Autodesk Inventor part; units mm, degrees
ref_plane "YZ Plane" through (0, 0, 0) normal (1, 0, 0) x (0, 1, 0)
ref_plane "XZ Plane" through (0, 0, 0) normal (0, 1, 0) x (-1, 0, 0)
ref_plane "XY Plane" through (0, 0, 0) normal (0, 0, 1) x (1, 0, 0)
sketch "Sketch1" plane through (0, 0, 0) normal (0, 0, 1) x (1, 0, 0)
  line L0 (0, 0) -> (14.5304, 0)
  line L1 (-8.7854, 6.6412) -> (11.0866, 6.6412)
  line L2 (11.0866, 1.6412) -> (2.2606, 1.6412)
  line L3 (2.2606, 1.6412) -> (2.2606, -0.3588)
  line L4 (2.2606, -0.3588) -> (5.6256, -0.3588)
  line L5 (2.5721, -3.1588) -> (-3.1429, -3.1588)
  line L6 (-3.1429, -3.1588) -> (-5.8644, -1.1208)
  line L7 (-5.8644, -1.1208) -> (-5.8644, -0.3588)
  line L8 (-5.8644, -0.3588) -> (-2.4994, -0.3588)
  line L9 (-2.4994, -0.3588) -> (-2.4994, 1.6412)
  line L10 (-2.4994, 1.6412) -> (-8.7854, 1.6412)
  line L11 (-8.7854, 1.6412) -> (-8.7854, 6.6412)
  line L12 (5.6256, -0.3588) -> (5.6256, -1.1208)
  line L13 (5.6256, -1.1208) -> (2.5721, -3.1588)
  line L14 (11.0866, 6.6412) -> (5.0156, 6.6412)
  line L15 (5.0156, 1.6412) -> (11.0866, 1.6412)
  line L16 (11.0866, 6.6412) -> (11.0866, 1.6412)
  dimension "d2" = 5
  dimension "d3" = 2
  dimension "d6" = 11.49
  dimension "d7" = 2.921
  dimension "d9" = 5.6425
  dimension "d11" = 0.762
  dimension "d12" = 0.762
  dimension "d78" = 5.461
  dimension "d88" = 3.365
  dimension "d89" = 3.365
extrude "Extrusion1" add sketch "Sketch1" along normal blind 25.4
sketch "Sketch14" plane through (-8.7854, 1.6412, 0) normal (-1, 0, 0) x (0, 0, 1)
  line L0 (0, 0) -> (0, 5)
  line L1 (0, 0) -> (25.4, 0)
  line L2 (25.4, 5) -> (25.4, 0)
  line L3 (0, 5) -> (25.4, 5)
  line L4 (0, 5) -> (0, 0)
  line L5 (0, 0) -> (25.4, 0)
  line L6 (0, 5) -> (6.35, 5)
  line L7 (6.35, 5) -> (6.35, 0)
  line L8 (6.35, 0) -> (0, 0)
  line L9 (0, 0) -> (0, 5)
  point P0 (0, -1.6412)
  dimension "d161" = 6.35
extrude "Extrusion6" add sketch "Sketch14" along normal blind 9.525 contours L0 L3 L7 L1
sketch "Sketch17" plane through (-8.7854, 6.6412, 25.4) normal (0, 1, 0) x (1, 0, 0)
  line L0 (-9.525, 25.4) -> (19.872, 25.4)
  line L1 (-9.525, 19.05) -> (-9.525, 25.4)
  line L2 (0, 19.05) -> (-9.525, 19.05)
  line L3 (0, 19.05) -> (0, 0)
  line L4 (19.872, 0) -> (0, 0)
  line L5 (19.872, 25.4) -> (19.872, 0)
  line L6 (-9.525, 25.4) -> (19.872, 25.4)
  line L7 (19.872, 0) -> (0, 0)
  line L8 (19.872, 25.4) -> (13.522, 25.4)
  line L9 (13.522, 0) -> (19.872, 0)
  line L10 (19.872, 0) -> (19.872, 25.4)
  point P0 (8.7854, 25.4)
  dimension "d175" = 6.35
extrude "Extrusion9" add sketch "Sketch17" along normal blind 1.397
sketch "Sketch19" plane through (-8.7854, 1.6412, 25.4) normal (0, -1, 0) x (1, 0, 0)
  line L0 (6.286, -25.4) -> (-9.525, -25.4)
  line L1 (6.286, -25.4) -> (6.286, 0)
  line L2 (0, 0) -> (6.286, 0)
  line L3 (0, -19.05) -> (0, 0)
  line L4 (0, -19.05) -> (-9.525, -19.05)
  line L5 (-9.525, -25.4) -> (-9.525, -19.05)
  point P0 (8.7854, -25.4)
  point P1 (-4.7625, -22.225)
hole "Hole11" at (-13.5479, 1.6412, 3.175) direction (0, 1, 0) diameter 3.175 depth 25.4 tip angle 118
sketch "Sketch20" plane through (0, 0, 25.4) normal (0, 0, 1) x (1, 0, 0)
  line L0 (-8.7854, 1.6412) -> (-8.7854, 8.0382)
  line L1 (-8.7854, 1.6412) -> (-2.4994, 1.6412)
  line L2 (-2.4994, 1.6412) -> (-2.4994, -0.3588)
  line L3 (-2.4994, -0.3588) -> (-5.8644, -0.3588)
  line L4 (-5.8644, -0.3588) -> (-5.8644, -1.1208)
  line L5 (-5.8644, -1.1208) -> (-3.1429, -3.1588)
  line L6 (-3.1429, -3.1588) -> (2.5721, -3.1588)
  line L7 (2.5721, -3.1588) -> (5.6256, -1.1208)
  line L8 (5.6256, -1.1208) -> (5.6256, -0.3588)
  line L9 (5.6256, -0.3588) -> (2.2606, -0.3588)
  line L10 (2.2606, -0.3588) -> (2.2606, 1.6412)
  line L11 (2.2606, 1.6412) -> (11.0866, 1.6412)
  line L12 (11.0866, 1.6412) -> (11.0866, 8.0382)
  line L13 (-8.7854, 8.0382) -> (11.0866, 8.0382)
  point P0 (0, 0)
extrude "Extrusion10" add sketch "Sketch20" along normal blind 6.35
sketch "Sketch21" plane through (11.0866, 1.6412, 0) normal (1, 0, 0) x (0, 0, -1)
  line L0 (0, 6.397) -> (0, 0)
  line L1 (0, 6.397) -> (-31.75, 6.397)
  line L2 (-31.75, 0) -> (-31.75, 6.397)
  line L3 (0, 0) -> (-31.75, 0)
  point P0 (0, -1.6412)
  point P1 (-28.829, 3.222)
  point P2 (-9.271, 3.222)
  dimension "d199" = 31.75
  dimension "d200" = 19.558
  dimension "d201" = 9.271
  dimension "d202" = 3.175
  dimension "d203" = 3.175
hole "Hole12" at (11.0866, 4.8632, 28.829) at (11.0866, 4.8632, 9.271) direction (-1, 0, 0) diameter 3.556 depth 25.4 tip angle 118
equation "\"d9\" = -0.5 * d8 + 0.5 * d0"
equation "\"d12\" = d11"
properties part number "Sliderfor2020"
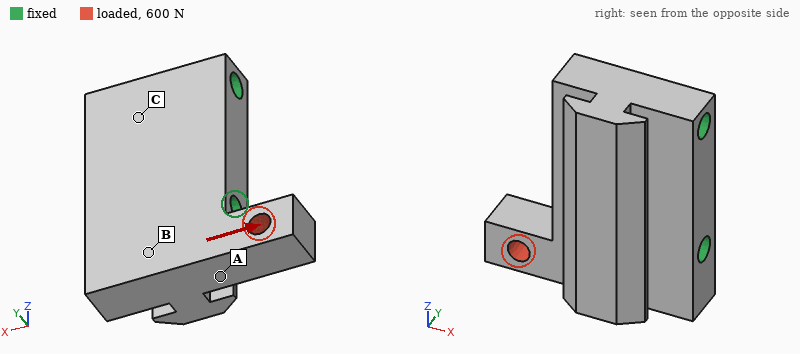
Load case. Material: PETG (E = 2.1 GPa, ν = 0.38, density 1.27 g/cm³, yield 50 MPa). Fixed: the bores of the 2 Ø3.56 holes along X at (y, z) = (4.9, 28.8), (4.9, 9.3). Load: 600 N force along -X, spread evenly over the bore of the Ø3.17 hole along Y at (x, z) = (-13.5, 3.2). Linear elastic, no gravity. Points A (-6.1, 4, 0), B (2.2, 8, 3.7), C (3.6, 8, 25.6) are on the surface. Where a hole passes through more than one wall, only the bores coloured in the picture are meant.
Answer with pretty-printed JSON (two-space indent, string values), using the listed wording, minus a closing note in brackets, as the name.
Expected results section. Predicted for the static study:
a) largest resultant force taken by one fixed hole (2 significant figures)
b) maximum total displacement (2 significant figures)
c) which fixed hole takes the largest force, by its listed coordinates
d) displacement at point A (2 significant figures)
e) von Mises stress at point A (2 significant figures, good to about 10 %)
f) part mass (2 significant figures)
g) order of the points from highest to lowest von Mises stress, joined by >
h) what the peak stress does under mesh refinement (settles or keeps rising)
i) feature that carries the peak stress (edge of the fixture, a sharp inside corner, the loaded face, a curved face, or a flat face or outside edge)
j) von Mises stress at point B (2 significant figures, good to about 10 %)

{
  "largest resultant force taken by one fixed hole": "610 N",
  "maximum total displacement": "0.19 mm",
  "which fixed hole takes the largest force, by its listed coordinates": "(4.9, 9.3)",
  "displacement at point A": "0.076 mm",
  "von Mises stress at point A": "17 MPa",
  "part mass": "6.5 g",
  "order of the points from highest to lowest von Mises stress, joined by >": "A > B > C",
  "what the peak stress does under mesh refinement": "keeps rising",
  "feature that carries the peak stress": "edge of the fixture",
  "von Mises stress at point B": "7.0 MPa"
}
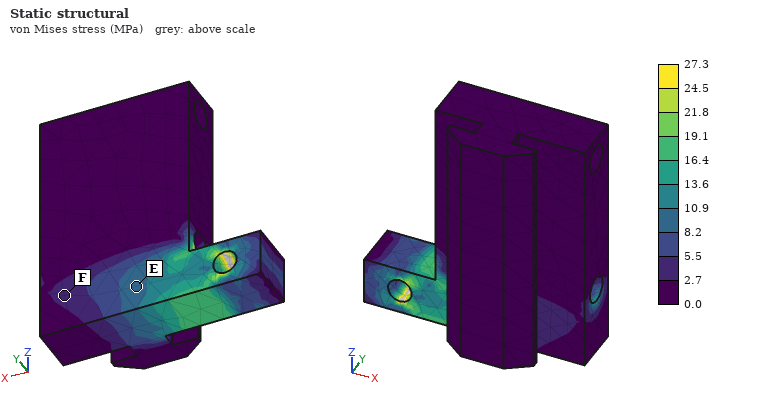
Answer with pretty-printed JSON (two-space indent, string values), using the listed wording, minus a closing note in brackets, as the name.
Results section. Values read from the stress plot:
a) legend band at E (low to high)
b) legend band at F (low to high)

{
  "legend band at E": "8.2 to 10.9 MPa",
  "legend band at F": "2.7 to 5.5 MPa"
}
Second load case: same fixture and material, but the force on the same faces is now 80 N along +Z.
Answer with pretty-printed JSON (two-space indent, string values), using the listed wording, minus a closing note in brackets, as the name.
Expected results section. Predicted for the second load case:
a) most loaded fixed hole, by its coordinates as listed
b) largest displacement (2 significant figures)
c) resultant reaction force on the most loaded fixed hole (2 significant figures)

{
  "most loaded fixed hole, by its coordinates as listed": "(4.9, 9.3)",
  "largest displacement": "0.13 mm",
  "resultant reaction force on the most loaded fixed hole": "80 N"
}
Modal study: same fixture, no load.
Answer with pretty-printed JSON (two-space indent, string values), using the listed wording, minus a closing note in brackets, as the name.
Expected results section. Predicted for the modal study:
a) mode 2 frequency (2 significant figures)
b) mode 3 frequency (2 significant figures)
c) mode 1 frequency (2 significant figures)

{
  "mode 2 frequency": "6800 Hz",
  "mode 3 frequency": "11 kHz",
  "mode 1 frequency": "5700 Hz"
}
